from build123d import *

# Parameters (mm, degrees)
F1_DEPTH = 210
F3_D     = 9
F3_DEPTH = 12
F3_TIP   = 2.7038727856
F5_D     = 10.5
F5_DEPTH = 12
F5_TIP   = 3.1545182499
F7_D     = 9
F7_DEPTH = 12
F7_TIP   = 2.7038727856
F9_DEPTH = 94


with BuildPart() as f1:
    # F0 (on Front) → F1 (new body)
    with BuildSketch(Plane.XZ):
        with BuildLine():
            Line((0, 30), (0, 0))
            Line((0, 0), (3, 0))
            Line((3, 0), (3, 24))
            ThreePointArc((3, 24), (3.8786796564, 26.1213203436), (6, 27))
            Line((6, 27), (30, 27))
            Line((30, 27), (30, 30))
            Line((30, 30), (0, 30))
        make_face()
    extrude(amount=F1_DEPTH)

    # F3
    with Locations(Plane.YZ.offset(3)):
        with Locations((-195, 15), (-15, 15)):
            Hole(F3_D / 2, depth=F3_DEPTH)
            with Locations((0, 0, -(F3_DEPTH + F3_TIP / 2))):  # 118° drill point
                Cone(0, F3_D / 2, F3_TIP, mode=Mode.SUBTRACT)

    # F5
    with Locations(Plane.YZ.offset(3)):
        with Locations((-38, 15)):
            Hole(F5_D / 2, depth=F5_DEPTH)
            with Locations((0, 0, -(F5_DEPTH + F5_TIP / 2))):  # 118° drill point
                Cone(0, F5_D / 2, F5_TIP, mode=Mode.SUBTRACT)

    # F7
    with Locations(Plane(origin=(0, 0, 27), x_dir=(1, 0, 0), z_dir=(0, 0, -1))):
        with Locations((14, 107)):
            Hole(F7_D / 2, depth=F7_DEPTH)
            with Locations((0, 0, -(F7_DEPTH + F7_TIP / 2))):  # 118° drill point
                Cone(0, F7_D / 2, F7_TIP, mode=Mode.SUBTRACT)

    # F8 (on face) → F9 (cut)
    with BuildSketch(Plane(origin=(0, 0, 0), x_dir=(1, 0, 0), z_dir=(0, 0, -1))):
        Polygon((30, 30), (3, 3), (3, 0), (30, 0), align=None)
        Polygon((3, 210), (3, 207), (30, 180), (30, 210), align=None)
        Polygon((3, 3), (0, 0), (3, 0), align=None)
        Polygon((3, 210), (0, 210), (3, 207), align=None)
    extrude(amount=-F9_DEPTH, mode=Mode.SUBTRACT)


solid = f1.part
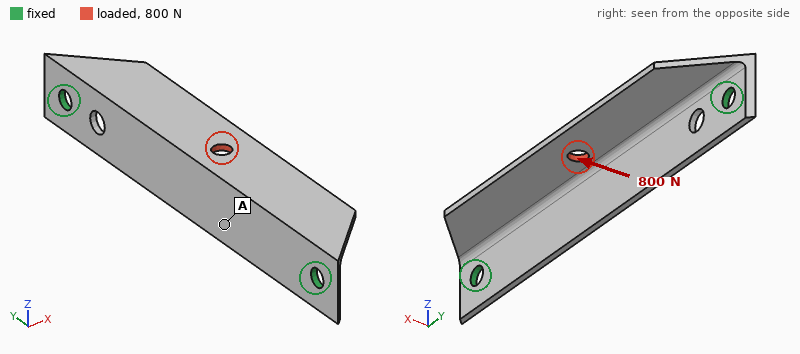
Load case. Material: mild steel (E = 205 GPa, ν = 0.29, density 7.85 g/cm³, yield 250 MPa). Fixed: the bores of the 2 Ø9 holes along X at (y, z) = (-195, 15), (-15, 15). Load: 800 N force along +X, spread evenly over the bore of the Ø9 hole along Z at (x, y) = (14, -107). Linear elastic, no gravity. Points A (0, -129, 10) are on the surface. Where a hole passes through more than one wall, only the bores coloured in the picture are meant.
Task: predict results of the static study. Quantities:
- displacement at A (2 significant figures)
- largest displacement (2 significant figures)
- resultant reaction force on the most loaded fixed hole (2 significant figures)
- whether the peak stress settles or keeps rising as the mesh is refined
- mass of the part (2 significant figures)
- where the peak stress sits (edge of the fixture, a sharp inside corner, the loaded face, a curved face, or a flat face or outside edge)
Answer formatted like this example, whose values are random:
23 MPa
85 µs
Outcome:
20 µm
75 µm
810 N
keeps rising
260 g
edge of the fixture
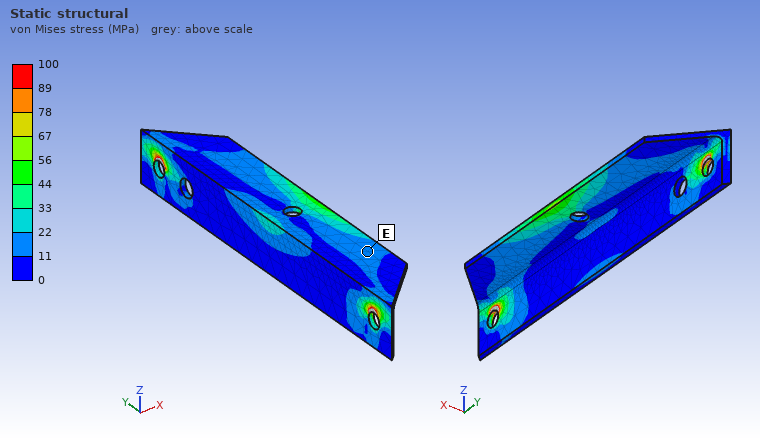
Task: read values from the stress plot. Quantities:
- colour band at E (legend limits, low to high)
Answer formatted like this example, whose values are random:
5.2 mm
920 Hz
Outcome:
11 to 22 MPa
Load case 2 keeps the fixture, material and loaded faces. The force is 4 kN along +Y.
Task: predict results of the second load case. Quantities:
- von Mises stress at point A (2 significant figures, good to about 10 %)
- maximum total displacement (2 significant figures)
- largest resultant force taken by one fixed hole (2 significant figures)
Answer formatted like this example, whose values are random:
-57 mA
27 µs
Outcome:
6.4 MPa
18 µm
2.1 kN
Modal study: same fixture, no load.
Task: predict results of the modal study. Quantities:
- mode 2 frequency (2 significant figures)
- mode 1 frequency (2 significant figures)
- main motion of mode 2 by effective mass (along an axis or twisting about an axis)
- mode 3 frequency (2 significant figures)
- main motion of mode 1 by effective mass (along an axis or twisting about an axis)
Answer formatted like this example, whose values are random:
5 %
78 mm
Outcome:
1700 Hz
980 Hz
along X
2000 Hz
along Z
